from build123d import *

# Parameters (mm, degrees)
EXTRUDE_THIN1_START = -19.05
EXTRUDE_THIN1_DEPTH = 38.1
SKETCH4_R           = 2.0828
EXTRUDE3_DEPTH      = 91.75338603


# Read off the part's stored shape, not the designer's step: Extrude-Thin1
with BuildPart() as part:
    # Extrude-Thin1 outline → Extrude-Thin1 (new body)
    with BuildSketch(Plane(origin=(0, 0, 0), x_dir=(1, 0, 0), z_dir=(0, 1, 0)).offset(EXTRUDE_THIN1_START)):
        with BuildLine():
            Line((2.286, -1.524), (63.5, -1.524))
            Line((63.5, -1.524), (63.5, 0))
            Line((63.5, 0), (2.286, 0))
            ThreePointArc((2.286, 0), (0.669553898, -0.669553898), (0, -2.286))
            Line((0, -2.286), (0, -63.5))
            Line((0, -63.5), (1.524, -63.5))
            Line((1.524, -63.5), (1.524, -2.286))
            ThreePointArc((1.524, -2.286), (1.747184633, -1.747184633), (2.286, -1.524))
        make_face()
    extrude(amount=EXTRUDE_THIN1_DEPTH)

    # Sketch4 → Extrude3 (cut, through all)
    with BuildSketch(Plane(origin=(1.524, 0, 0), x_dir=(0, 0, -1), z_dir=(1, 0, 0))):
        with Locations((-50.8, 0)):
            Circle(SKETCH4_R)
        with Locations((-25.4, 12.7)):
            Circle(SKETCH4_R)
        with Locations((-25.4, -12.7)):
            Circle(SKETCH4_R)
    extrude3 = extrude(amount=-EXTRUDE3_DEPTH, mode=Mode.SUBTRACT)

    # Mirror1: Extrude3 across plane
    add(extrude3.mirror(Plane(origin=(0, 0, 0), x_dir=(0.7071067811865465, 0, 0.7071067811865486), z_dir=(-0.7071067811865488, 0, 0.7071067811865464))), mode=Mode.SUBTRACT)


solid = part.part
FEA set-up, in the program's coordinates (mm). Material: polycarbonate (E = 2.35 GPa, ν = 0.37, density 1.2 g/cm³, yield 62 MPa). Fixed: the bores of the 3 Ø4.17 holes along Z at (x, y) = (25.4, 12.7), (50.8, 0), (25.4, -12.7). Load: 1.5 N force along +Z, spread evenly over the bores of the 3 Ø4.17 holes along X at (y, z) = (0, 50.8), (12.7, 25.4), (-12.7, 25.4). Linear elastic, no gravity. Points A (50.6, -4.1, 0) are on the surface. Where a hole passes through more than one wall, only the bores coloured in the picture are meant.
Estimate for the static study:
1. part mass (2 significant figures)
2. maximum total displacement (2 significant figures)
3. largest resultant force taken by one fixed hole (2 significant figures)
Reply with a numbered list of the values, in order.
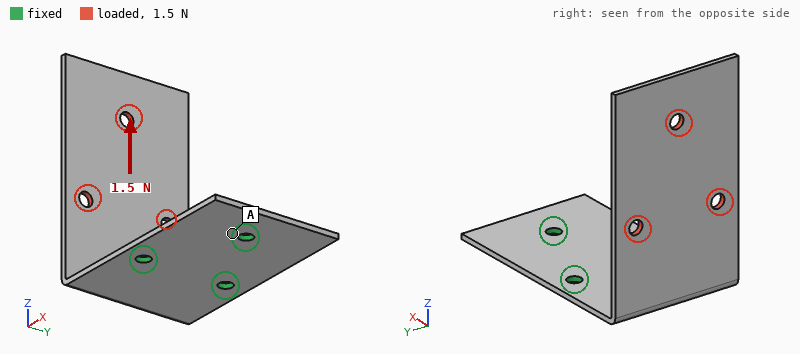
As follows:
1. 8.5 g
2. 0.98 mm
3. 0.83 N
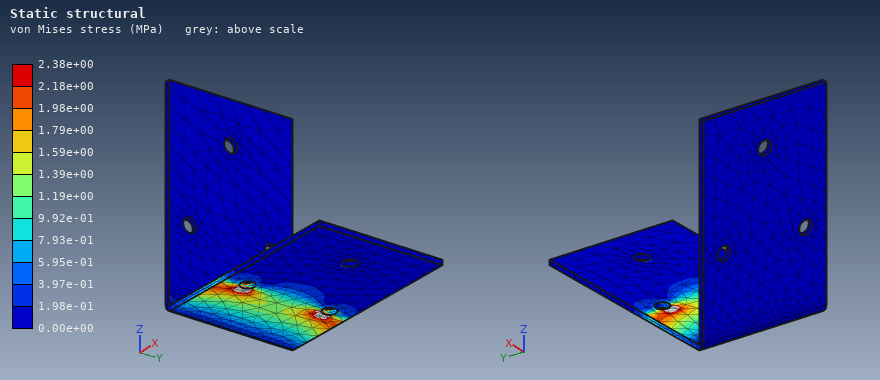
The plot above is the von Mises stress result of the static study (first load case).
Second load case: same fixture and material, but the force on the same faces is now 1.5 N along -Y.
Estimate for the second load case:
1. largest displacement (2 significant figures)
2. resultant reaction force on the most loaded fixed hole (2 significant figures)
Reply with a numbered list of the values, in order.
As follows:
1. 0.94 mm
2. 2.3 N
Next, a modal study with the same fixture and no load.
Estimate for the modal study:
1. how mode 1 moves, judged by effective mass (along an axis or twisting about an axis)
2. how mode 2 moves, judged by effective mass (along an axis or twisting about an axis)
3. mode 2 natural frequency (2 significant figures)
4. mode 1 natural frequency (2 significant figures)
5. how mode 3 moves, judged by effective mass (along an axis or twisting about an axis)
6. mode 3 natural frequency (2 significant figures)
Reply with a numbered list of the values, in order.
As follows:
1. along X
2. along Y
3. 120 Hz
4. 57 Hz
5. along Z
6. 240 Hz
